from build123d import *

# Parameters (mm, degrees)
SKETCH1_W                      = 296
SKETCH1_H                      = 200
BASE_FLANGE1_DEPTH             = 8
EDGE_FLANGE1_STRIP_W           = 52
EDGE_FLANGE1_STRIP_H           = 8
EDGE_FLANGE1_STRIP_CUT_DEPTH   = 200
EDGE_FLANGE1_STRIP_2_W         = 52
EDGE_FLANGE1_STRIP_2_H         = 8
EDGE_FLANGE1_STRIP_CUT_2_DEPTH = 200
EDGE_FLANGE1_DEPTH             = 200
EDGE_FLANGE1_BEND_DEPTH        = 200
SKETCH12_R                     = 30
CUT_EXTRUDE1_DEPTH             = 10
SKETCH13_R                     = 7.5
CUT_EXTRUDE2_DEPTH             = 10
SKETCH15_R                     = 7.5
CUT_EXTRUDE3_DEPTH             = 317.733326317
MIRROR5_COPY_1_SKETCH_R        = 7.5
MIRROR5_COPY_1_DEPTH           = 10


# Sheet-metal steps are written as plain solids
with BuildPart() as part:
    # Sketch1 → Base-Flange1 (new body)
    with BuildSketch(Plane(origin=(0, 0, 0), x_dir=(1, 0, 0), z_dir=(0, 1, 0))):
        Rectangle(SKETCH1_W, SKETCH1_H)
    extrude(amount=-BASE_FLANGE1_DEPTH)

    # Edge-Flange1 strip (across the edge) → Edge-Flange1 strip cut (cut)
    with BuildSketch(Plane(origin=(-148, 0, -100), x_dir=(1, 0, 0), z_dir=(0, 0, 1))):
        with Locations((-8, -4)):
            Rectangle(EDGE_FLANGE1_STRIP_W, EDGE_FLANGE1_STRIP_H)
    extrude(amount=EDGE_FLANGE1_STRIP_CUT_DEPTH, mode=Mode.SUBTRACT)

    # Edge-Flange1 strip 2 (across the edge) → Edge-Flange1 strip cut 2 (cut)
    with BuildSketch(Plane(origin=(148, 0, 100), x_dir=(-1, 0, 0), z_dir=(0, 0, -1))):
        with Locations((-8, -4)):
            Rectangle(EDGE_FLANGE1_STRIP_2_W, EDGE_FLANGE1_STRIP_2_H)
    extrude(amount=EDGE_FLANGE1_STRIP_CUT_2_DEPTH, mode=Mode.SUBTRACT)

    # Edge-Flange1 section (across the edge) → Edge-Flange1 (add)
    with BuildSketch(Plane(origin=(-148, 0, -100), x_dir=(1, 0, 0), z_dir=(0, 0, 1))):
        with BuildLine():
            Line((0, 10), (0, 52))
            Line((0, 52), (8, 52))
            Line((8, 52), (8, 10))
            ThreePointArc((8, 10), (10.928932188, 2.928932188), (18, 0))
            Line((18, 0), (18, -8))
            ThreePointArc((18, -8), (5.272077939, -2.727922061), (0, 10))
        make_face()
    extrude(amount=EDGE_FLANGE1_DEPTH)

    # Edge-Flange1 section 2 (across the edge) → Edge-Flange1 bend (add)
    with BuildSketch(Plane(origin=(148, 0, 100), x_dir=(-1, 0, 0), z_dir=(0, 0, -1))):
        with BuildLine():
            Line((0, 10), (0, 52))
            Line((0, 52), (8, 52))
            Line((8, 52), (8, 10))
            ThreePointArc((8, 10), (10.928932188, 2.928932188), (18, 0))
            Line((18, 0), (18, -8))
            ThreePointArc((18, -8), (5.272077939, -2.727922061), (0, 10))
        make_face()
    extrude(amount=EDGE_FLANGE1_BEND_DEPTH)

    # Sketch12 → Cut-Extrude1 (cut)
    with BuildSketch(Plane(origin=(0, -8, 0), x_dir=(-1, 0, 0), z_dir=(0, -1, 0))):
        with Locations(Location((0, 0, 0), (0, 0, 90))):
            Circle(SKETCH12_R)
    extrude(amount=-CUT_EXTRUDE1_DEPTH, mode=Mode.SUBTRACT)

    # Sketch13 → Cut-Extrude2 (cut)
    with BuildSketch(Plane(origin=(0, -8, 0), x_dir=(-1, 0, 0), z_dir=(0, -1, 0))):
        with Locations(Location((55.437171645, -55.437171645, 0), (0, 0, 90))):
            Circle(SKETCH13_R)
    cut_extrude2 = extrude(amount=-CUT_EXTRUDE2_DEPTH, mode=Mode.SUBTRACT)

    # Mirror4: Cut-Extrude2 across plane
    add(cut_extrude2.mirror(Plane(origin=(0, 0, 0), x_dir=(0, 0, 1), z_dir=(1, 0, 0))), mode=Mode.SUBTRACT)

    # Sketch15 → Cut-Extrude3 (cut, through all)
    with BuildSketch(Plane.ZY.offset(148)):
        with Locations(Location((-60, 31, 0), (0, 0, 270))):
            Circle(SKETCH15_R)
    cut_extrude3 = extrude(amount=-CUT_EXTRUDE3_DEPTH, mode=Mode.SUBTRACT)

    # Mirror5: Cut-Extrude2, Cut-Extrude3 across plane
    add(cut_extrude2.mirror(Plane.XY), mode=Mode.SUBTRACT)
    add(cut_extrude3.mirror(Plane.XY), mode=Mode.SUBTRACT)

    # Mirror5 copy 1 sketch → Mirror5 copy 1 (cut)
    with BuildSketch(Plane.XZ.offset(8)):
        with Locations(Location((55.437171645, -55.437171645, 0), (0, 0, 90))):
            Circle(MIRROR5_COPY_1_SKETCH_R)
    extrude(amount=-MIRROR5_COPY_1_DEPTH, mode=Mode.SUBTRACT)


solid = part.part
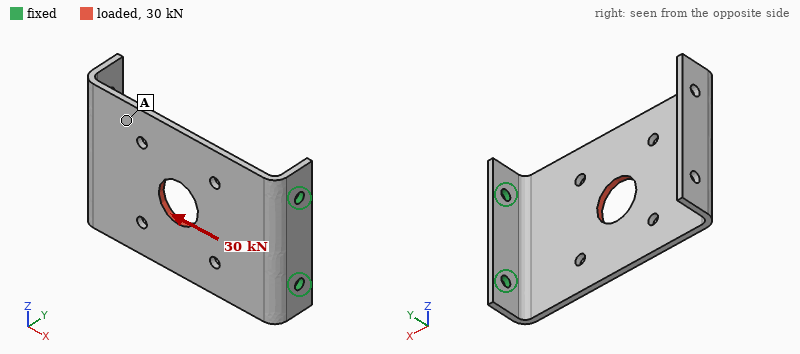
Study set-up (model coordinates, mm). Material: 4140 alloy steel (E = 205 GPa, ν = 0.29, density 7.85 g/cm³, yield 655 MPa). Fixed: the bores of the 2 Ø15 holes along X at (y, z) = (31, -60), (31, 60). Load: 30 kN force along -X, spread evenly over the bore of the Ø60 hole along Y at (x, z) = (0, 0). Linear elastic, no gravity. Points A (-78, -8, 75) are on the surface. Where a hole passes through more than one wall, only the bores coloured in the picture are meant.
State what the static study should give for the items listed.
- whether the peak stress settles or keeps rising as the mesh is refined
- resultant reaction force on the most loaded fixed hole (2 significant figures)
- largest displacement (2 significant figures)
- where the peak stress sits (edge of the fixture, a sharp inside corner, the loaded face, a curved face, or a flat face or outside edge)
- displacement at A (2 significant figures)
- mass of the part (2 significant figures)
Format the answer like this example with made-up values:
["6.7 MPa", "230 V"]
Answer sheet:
["keeps rising", "15 kN", "3.3 mm", "edge of the fixture", "2.5 mm", "4.6 kg"]
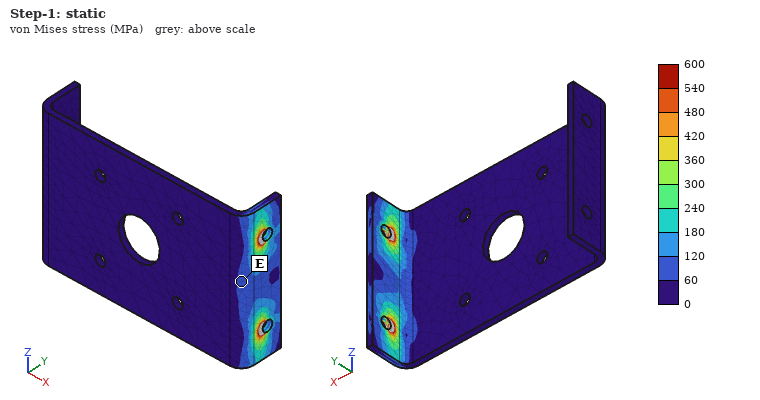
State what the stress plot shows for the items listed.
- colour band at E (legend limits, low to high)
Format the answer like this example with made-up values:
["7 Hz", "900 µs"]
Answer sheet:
["60 to 120 MPa"]
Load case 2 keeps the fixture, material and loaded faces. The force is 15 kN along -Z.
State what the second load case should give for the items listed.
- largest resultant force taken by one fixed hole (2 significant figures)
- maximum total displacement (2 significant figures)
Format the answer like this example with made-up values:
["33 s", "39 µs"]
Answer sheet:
["19 kN", "1.5 mm"]
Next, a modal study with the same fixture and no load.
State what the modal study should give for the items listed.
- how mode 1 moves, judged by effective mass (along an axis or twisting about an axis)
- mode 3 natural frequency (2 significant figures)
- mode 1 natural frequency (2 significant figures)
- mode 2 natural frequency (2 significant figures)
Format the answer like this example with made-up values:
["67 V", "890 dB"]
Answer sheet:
["along Y", "330 Hz", "52 Hz", "180 Hz"]
